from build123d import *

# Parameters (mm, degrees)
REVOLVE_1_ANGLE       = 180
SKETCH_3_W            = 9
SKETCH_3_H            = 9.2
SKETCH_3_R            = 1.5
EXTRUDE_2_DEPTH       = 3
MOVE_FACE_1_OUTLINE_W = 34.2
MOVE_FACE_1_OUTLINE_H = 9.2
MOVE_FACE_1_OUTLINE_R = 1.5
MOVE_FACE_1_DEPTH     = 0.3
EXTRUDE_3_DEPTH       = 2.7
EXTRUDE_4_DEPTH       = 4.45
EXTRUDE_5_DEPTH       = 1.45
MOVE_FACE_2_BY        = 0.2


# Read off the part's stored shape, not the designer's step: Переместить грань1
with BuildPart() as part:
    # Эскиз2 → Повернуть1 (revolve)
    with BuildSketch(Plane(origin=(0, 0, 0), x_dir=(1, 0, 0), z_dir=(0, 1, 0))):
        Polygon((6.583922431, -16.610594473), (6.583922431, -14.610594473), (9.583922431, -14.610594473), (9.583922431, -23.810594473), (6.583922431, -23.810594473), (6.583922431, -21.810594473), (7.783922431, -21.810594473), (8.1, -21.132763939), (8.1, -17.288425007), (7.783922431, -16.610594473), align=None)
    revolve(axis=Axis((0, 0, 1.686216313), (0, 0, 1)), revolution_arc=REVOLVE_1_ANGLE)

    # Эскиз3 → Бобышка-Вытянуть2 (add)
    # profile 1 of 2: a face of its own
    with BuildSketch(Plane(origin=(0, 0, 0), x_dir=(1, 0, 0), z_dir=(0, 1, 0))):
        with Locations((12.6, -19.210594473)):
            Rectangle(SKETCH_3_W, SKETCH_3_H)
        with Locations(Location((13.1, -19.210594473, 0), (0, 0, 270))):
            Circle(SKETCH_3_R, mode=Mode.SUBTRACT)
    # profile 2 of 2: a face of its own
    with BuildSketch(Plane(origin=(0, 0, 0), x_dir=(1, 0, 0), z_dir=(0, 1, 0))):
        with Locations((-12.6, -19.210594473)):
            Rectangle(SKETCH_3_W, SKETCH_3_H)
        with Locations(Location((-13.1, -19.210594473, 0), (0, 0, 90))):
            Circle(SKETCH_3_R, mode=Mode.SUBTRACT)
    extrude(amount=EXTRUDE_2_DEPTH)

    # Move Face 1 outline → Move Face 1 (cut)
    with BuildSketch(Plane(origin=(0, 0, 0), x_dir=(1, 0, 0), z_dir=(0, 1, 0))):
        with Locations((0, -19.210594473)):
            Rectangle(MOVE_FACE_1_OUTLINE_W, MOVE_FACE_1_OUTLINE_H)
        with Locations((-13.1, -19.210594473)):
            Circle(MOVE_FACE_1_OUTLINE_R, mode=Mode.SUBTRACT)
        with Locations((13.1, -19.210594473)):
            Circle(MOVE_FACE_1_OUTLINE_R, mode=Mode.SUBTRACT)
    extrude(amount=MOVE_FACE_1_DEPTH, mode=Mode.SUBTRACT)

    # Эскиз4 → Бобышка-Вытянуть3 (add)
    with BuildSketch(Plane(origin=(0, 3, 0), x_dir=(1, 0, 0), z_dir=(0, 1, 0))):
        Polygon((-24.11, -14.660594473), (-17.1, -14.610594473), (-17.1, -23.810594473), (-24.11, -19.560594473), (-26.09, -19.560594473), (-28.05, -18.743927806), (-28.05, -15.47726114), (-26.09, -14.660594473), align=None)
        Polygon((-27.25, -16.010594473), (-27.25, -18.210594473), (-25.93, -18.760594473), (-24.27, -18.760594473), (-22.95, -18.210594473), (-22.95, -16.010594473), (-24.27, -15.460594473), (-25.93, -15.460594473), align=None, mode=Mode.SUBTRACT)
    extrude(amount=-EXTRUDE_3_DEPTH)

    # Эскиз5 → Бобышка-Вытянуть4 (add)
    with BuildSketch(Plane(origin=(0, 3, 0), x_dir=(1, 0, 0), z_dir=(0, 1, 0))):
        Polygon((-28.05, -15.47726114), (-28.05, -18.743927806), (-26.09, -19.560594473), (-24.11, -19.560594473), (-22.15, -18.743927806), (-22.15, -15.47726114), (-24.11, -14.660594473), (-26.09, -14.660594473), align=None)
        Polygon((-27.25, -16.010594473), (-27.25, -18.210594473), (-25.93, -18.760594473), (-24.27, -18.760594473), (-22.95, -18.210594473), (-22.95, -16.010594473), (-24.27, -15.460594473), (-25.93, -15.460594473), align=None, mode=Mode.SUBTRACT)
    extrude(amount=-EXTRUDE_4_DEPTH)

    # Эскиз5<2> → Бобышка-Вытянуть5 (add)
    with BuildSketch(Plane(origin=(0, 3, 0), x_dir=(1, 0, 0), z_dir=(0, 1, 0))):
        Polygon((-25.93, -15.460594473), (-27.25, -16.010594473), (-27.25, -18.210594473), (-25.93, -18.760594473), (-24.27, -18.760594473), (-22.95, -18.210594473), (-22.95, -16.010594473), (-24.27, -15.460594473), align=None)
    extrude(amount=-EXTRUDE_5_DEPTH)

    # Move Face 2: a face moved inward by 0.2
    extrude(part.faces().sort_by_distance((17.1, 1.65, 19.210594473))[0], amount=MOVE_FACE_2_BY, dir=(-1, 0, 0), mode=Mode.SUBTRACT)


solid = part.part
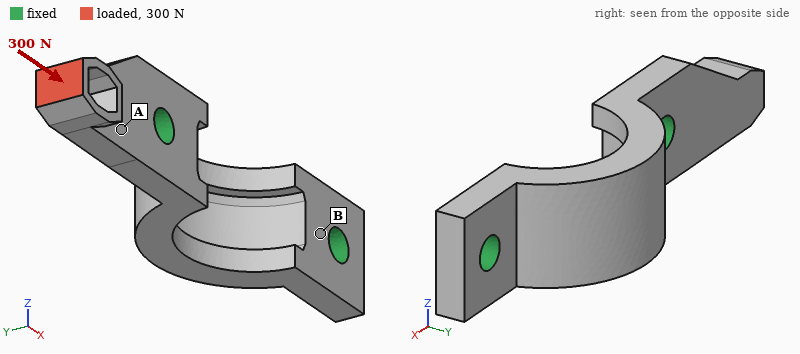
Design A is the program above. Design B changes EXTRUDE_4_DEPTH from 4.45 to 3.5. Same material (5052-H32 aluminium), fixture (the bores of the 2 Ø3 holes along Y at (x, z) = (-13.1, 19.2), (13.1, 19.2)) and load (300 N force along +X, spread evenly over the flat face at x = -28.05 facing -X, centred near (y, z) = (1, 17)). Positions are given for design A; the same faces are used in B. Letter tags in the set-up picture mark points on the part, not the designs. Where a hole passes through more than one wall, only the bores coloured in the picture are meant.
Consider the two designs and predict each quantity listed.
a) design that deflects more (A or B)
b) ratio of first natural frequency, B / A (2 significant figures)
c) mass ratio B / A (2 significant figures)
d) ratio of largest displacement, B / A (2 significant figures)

A
1.1
0.99
0.64
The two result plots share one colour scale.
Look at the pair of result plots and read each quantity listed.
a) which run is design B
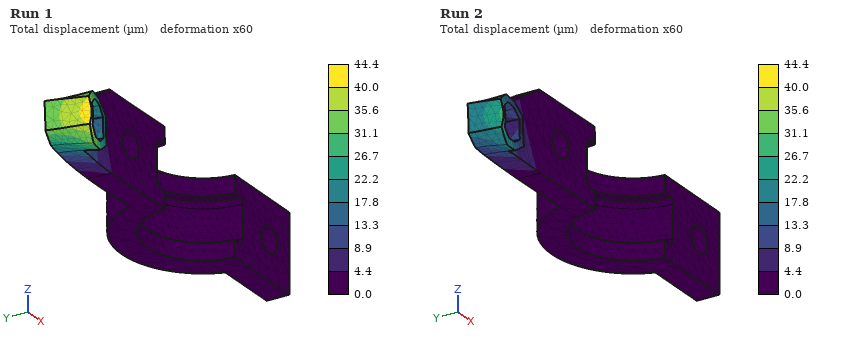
Run 2
